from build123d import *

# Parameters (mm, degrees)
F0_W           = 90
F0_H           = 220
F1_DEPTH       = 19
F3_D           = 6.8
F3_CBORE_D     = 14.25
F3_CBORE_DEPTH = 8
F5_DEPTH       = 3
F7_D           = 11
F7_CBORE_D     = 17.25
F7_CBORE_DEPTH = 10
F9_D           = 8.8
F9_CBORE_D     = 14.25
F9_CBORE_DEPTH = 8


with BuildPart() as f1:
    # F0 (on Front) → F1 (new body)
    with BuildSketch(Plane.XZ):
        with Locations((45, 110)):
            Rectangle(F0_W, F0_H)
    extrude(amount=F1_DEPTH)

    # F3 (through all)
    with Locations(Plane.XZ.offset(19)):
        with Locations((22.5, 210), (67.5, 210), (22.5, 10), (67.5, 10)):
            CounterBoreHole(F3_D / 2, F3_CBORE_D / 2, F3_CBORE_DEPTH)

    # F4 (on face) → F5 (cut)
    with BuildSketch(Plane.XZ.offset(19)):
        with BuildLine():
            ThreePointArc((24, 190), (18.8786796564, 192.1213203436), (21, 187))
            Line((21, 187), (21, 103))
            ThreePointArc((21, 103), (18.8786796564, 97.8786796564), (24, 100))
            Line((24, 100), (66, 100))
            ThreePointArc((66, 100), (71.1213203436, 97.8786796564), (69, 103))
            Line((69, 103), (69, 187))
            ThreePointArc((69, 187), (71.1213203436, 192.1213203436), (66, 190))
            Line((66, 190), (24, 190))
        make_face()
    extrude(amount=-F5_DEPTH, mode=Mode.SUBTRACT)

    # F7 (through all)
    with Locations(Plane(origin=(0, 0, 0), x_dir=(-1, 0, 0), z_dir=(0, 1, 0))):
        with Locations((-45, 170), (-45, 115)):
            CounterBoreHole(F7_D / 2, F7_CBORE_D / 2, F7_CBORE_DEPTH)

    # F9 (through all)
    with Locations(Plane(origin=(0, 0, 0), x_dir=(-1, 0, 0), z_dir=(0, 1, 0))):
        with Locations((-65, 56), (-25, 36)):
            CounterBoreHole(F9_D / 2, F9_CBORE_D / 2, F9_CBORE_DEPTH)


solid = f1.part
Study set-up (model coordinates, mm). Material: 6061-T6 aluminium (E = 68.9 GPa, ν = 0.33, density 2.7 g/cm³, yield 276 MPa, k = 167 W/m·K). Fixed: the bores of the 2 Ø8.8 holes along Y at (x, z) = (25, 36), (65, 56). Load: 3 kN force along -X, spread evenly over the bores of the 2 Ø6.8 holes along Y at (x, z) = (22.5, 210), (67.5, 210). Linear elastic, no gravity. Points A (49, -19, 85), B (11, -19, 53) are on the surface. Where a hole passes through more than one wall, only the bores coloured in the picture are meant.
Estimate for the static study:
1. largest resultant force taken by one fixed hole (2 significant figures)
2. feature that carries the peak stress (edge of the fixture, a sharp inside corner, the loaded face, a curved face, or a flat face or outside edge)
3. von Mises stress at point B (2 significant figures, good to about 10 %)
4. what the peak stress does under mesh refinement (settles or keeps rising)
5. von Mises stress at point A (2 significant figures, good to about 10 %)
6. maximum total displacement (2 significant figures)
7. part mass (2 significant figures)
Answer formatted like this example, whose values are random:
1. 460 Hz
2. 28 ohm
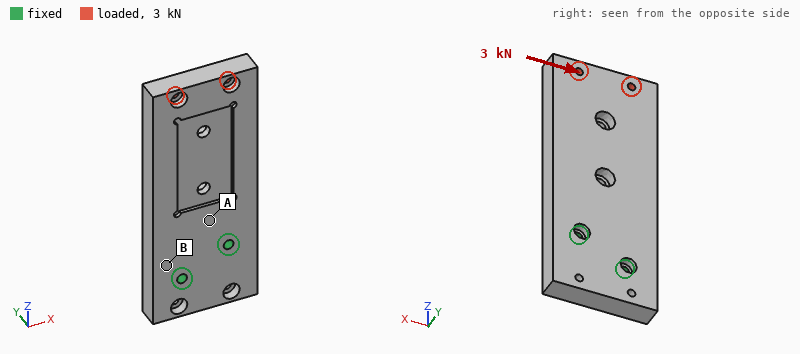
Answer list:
1. 11 kN
2. edge of the fixture
3. 17 MPa
4. keeps rising
5. 7.5 MPa
6. 0.13 mm
7. 940 g
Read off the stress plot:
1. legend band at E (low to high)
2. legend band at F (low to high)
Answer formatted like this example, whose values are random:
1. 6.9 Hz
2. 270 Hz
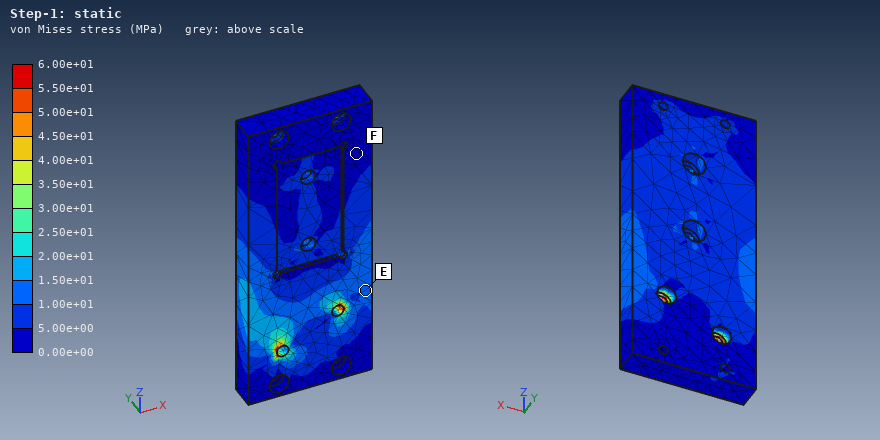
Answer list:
1. 1.00e+01 to 1.50e+01 MPa
2. 0.00e+00 to 5.00e+00 MPa
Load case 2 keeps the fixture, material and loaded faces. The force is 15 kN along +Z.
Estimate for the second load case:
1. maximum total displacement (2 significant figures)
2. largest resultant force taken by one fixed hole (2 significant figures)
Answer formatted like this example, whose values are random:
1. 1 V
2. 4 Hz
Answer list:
1. 0.40 mm
2. 7.6 kN
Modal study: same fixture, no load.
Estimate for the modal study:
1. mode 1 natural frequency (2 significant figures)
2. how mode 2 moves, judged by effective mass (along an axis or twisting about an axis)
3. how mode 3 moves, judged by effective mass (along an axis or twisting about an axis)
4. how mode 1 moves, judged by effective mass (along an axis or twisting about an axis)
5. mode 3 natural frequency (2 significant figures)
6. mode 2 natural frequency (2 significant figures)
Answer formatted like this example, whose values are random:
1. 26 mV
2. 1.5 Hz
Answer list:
1. 450 Hz
2. along X
3. along X
4. along Y
5. 1700 Hz
6. 1600 Hz
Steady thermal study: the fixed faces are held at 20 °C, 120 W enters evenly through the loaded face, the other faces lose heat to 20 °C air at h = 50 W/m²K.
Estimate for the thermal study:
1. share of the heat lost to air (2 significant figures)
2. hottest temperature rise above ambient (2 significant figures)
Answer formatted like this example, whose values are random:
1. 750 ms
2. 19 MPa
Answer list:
1. 48 %
2. 59 K
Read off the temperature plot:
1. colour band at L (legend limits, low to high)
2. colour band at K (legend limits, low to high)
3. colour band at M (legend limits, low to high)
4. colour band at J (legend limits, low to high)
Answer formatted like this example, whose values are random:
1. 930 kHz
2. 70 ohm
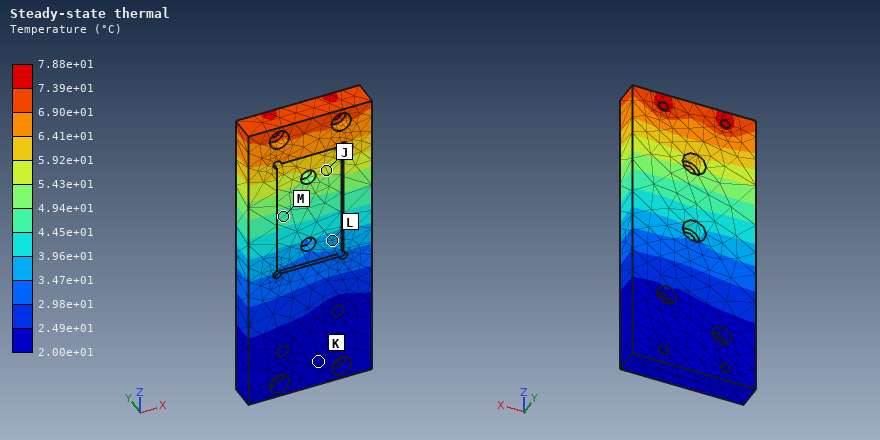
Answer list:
1. 3.47e+01 to 3.96e+01 °C
2. 2.00e+01 to 2.49e+01 °C
3. 4.45e+01 to 4.94e+01 °C
4. 5.43e+01 to 5.92e+01 °C
